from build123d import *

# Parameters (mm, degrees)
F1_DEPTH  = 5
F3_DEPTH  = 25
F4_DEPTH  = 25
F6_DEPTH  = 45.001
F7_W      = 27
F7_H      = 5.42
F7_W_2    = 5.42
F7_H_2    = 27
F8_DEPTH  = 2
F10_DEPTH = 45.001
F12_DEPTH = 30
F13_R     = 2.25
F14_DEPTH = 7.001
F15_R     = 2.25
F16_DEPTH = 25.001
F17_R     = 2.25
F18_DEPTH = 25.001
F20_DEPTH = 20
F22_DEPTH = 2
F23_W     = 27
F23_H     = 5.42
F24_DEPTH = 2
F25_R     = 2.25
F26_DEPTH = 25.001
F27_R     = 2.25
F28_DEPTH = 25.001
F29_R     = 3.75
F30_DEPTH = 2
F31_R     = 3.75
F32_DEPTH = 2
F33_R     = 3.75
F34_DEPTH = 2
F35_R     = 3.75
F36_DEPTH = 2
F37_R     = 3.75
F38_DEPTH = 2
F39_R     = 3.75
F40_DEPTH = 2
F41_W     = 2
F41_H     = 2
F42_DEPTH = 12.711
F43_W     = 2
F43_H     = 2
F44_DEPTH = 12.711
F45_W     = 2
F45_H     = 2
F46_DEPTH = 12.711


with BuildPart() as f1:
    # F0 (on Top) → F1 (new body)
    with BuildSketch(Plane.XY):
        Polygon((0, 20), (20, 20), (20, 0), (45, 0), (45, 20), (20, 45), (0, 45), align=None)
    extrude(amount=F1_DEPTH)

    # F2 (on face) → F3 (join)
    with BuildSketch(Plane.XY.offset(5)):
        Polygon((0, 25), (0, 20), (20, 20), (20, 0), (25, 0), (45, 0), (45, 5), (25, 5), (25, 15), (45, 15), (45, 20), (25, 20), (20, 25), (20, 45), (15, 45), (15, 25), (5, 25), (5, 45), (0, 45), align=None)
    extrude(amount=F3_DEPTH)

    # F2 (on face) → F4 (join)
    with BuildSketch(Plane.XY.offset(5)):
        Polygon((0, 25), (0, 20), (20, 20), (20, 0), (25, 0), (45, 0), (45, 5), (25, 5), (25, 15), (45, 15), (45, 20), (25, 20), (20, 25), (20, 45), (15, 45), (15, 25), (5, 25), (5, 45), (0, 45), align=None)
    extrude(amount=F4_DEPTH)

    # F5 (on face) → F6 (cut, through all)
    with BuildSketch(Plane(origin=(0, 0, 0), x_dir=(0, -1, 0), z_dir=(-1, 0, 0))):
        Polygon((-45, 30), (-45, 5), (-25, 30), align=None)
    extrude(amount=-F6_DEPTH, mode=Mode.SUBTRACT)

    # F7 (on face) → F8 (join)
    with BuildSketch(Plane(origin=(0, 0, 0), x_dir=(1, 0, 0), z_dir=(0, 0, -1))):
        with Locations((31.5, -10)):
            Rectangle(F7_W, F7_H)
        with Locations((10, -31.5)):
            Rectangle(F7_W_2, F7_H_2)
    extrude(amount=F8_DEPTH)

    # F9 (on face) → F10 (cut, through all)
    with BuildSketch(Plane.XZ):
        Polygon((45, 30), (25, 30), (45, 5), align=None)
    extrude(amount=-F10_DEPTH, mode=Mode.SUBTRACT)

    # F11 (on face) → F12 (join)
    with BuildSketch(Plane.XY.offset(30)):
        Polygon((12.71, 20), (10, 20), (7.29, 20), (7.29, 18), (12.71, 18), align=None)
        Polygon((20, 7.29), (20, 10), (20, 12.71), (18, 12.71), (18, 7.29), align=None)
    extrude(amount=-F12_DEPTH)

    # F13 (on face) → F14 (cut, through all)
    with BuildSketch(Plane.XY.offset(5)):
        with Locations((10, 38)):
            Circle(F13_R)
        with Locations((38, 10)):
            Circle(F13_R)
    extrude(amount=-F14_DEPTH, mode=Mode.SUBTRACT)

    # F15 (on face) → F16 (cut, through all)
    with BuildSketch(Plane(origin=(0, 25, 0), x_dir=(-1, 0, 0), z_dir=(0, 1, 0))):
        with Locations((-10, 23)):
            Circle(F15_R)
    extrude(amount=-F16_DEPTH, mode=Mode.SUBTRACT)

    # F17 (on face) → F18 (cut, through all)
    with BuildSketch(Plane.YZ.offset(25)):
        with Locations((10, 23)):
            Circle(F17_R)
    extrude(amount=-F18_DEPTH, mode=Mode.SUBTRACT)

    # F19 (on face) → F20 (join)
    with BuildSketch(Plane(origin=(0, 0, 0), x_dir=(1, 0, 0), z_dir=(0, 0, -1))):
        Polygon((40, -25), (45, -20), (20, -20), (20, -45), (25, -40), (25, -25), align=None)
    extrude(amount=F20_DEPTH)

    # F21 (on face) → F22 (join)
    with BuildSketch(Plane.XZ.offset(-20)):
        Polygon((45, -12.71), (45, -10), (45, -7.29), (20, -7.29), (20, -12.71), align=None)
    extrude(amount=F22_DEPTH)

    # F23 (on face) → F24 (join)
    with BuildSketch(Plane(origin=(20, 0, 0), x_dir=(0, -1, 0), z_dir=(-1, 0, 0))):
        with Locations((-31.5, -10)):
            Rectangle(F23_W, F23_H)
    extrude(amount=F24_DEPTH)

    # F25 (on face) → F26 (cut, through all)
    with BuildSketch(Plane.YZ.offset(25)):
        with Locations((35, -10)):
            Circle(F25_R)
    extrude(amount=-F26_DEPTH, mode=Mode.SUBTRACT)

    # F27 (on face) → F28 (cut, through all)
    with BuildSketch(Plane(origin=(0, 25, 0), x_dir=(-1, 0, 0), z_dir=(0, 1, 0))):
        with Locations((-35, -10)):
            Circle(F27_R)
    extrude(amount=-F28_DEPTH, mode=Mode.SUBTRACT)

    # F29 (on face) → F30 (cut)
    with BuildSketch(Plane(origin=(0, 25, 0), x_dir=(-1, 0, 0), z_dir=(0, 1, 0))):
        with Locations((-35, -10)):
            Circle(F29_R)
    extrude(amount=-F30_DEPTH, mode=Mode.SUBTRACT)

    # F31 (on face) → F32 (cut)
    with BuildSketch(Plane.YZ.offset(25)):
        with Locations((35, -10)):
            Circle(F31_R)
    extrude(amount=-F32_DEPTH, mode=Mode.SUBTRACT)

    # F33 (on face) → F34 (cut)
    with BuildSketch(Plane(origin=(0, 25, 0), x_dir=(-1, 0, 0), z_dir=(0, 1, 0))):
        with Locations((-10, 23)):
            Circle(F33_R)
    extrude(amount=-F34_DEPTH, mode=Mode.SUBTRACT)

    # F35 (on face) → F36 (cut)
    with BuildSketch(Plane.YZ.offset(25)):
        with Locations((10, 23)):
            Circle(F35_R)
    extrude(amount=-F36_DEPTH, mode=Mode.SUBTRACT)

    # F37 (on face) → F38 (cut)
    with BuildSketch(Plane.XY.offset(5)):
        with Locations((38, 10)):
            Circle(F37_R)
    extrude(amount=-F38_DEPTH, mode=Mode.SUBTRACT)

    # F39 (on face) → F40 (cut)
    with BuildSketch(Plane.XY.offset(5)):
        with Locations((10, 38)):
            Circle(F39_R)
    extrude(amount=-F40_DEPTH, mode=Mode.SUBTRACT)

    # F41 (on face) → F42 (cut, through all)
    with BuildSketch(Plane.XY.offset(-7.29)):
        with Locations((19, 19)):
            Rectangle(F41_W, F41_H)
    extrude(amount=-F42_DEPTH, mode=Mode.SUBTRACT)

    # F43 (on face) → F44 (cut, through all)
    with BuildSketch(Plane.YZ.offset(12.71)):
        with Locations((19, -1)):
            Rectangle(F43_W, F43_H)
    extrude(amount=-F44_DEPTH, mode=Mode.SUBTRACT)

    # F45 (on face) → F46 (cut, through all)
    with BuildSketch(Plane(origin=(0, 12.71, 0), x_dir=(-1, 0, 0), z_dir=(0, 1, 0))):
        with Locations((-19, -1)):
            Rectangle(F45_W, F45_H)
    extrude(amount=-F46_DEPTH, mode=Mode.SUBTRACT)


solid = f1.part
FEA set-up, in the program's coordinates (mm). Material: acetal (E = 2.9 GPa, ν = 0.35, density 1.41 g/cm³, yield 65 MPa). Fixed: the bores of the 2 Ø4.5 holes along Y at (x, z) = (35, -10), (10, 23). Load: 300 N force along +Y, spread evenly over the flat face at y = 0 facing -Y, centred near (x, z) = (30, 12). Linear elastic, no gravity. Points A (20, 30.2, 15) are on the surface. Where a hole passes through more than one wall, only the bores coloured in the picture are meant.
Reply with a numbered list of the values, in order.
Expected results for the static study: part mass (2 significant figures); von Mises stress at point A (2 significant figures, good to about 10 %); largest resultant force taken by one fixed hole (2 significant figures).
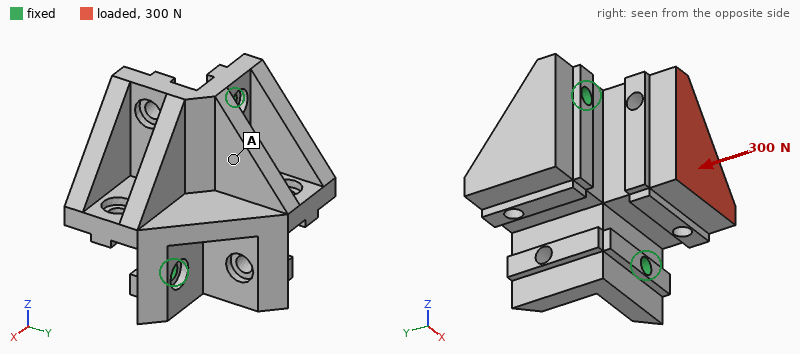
1. 30 g
2. 2.9 MPa
3. 160 N
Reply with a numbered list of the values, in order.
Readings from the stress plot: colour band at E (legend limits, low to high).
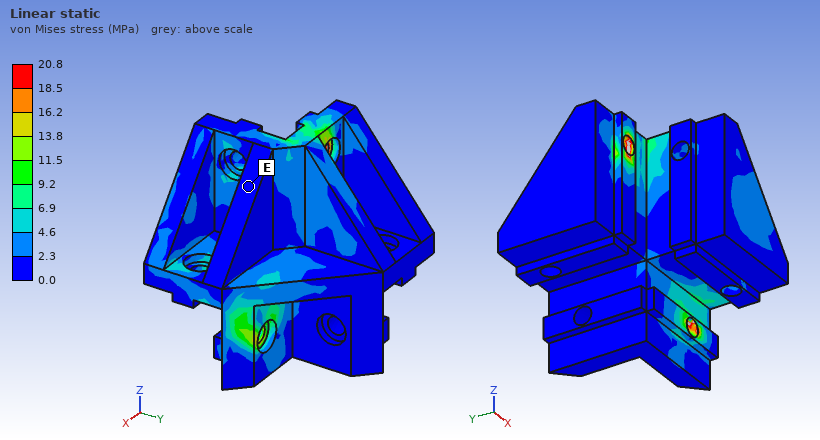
1. 0.0 to 2.3 MPa
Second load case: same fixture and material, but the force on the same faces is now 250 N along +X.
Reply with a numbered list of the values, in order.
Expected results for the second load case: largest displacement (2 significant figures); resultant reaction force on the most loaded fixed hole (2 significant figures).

1. 0.69 mm
2. 170 N
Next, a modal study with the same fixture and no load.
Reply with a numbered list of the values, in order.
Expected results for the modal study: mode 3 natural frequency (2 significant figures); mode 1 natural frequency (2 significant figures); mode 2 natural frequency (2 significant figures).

1. 2600 Hz
2. 1000 Hz
3. 2100 Hz
